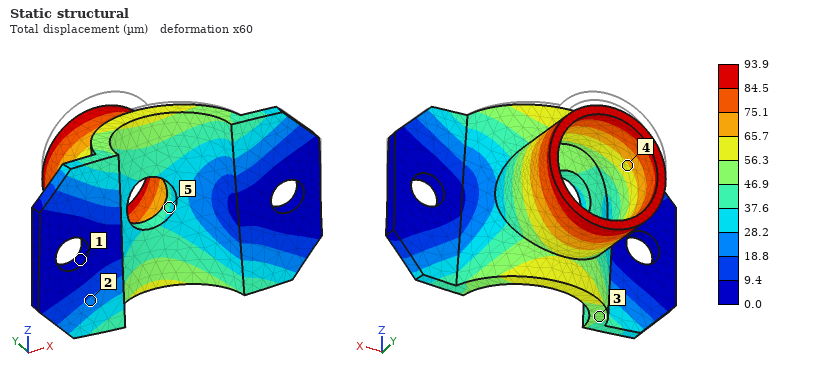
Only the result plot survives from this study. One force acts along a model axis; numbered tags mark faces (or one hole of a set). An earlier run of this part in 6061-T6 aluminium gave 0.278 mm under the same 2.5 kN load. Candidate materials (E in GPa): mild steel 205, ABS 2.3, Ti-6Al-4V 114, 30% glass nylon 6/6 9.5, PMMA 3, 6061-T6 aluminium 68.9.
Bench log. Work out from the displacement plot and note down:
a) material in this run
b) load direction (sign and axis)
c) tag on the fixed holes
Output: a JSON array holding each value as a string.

["mild steel", "-Z", "1"]
